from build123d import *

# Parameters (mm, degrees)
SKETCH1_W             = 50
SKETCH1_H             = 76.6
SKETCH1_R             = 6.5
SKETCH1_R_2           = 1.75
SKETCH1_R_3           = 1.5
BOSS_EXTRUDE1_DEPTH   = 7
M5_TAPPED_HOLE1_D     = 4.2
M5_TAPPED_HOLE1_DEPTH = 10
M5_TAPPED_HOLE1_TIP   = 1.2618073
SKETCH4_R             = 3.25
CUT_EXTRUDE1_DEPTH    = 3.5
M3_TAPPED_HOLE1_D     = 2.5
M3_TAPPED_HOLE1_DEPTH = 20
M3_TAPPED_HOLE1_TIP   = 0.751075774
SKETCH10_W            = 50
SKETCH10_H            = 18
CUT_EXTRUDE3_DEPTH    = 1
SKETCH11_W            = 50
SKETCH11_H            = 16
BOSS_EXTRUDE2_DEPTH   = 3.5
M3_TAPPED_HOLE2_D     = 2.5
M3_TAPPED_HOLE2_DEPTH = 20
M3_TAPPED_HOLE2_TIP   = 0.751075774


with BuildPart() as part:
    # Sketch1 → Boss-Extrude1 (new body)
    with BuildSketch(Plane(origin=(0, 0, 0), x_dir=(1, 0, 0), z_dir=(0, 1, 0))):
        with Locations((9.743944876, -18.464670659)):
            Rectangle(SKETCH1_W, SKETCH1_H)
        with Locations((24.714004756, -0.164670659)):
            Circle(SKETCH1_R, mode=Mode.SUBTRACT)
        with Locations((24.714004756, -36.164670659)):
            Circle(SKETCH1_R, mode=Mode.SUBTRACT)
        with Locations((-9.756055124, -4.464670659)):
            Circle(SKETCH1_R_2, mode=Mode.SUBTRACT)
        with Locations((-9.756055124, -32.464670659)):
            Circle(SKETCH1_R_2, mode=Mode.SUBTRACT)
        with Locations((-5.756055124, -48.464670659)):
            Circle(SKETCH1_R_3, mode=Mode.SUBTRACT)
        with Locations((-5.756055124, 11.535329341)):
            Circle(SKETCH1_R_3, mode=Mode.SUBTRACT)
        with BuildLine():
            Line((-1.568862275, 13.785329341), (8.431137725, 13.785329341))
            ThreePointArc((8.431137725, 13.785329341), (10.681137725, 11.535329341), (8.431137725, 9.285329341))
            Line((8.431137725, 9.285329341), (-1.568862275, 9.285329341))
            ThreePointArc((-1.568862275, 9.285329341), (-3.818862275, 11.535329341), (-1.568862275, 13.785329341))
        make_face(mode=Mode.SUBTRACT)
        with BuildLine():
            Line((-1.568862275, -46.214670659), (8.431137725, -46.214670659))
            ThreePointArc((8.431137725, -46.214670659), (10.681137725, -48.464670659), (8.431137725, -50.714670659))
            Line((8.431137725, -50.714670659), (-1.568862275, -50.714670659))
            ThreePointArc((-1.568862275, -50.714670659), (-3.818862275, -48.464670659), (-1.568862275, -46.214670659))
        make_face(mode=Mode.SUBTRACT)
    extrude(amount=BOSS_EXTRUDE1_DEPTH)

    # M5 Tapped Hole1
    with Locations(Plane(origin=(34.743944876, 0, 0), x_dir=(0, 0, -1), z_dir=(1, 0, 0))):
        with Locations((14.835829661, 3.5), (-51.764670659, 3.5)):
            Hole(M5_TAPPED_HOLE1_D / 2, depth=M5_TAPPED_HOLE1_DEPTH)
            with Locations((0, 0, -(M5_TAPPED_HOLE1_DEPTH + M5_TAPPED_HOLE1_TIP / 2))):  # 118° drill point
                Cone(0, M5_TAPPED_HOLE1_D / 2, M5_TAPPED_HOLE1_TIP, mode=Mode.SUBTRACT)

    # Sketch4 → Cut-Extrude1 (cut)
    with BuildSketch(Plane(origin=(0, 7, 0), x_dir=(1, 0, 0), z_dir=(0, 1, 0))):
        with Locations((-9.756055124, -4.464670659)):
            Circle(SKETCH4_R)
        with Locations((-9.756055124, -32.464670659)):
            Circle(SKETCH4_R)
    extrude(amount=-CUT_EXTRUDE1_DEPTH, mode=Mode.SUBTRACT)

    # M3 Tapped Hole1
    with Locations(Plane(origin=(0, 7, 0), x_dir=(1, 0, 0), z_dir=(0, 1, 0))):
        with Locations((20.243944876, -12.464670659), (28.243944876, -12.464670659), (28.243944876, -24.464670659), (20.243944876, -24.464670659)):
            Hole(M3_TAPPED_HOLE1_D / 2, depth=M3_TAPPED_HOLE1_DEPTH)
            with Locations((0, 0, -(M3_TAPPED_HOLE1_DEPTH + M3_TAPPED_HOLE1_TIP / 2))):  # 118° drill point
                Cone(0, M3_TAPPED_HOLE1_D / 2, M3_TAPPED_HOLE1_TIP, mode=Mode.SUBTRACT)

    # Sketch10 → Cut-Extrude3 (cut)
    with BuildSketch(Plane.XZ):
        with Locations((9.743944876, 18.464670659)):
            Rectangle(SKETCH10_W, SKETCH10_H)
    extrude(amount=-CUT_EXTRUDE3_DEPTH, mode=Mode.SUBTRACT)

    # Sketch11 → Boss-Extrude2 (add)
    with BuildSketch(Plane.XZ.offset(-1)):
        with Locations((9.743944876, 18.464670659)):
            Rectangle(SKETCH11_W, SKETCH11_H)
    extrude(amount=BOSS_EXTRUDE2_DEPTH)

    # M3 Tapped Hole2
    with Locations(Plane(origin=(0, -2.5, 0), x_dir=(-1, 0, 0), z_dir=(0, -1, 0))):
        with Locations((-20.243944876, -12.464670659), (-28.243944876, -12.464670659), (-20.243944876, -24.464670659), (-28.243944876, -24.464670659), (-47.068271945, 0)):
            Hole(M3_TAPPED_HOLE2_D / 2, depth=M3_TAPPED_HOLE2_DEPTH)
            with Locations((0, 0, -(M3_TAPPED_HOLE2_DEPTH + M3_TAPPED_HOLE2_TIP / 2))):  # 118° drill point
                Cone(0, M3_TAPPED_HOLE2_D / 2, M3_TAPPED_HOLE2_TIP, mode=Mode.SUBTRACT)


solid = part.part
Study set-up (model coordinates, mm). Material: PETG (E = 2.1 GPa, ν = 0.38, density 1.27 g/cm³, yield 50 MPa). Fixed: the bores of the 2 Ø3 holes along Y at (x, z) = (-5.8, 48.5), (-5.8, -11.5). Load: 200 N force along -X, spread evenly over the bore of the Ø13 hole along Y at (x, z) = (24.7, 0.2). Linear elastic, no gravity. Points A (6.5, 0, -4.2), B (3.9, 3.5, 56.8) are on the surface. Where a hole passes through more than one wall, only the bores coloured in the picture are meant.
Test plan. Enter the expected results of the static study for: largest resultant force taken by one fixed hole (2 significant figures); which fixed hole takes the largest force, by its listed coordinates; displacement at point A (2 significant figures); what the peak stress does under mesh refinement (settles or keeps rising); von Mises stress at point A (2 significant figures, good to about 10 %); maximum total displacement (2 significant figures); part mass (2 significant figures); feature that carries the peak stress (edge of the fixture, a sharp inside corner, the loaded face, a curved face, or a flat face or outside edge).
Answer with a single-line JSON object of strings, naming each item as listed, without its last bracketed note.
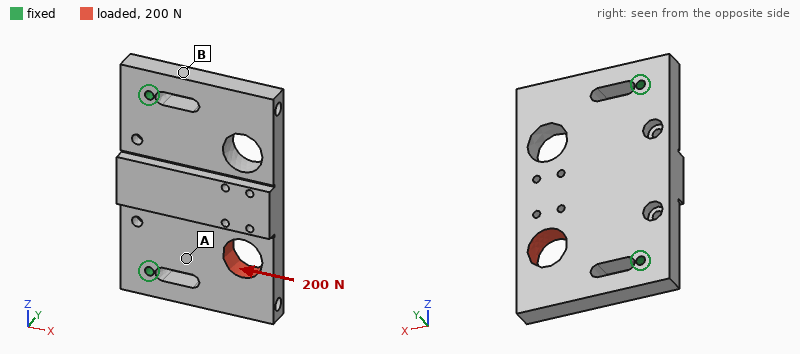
{"largest resultant force taken by one fixed hole": "160 N", "which fixed hole takes the largest force, by its listed coordinates": "(-5.8, -11.5)", "displacement at point A": "17 µm", "what the peak stress does under mesh refinement": "keeps rising", "von Mises stress at point A": "1.3 MPa", "maximum total displacement": "41 µm", "part mass": "32 g", "feature that carries the peak stress": "edge of the fixture"}
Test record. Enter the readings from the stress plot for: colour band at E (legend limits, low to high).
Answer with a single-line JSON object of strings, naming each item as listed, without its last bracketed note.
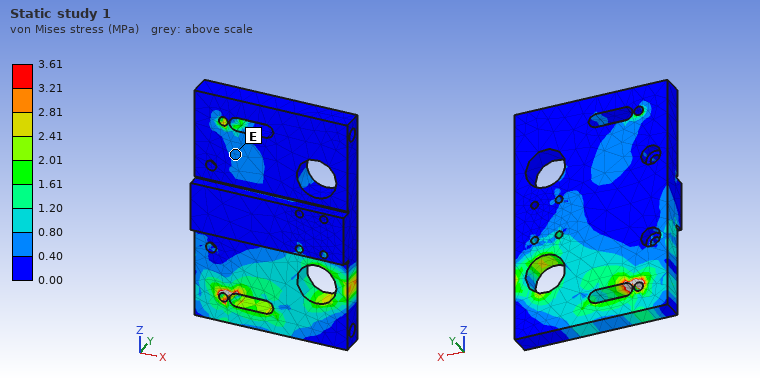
{"colour band at E": "0.40 to 0.80 MPa"}
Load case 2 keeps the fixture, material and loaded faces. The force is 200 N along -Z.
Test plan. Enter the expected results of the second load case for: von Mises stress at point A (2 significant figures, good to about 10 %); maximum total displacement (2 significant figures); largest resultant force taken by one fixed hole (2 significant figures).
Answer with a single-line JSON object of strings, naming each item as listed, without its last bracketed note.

{"von Mises stress at point A": "0.94 MPa", "maximum total displacement": "60 µm", "largest resultant force taken by one fixed hole": "140 N"}
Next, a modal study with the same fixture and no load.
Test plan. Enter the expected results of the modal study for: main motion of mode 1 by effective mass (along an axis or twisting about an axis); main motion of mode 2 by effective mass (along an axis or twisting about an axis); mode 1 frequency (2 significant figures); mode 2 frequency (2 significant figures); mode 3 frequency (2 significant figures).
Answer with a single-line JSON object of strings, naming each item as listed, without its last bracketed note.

{"main motion of mode 1 by effective mass": "along Y", "main motion of mode 2 by effective mass": "twisting about X", "mode 1 frequency": "540 Hz", "mode 2 frequency": "1200 Hz", "mode 3 frequency": "1800 Hz"}
